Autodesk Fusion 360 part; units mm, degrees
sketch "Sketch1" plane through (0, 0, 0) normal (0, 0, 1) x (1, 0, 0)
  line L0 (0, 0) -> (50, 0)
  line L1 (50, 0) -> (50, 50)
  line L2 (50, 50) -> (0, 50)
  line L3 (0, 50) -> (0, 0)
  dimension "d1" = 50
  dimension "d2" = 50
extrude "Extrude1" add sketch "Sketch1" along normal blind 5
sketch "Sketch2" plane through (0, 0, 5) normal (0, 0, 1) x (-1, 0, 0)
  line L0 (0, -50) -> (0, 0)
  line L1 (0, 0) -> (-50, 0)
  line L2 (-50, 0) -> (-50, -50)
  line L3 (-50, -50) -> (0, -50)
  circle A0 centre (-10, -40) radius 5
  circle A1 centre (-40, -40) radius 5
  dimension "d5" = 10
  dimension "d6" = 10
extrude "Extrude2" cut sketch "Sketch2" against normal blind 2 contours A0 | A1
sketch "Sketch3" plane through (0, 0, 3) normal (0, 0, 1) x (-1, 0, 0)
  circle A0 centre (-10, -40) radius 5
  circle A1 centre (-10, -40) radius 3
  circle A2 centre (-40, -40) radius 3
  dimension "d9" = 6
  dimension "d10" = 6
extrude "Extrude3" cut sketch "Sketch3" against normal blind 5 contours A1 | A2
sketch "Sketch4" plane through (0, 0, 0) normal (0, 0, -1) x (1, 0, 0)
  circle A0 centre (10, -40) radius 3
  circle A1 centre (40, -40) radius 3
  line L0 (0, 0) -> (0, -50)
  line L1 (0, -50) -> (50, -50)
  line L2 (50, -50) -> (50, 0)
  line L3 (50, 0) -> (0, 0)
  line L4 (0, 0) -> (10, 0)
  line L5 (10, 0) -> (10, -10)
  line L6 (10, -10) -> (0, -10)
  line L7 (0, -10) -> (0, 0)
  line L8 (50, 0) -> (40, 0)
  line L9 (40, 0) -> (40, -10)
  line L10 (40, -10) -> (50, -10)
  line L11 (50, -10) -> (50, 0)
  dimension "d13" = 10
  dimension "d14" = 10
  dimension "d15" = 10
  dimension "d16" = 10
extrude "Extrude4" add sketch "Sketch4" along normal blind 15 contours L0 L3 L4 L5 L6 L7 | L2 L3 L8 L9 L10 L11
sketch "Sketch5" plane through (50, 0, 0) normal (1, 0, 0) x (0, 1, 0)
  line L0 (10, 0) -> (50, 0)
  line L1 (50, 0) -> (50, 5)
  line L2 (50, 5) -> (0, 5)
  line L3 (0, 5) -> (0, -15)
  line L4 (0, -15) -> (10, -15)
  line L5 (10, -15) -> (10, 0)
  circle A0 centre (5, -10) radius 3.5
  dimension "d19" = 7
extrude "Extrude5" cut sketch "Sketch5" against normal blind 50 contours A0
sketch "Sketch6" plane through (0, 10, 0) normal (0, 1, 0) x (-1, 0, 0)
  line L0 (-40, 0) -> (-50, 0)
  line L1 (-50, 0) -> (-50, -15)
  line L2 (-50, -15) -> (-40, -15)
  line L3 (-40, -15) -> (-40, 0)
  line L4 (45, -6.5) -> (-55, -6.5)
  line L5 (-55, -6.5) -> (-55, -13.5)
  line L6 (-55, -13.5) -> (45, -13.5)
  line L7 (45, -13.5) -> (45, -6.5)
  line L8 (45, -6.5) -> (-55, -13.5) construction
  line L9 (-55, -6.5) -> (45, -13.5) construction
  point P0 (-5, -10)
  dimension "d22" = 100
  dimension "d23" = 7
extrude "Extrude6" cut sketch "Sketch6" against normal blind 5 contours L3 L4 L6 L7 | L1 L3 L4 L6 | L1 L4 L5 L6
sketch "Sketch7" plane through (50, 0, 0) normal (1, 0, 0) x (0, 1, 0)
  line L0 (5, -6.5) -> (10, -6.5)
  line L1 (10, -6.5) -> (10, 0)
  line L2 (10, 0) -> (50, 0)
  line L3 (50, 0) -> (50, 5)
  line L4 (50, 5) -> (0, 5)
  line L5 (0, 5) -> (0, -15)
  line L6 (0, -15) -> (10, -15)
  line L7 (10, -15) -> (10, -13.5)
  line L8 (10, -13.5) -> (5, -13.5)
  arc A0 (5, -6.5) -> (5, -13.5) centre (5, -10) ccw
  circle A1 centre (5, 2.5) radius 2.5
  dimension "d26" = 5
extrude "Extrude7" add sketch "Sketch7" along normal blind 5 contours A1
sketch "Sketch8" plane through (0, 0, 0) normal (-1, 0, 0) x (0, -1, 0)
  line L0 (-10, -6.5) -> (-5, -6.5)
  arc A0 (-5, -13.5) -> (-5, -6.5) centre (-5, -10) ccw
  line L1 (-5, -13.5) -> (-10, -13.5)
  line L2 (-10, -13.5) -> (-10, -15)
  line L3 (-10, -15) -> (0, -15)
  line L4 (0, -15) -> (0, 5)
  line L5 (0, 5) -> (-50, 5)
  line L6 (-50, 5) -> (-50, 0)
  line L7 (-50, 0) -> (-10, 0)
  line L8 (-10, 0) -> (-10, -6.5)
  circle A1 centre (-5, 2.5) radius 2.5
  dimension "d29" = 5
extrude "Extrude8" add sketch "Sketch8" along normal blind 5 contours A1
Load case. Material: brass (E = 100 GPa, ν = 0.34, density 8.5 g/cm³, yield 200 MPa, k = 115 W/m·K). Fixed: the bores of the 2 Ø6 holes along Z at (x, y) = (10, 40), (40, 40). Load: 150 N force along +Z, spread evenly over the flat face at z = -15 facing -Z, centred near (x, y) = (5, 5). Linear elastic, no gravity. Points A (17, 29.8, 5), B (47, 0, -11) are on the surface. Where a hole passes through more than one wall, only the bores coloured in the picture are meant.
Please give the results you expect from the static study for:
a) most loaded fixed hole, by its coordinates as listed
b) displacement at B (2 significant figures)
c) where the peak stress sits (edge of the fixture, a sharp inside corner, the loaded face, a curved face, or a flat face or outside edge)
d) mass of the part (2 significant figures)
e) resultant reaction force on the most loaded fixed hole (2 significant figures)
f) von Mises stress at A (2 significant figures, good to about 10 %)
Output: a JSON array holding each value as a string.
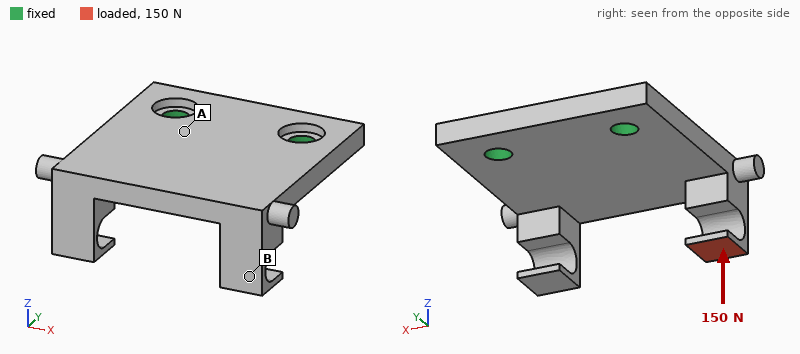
["(10, 40)", "0.050 mm", "a curved face", "120 g", "160 N", "23 MPa"]
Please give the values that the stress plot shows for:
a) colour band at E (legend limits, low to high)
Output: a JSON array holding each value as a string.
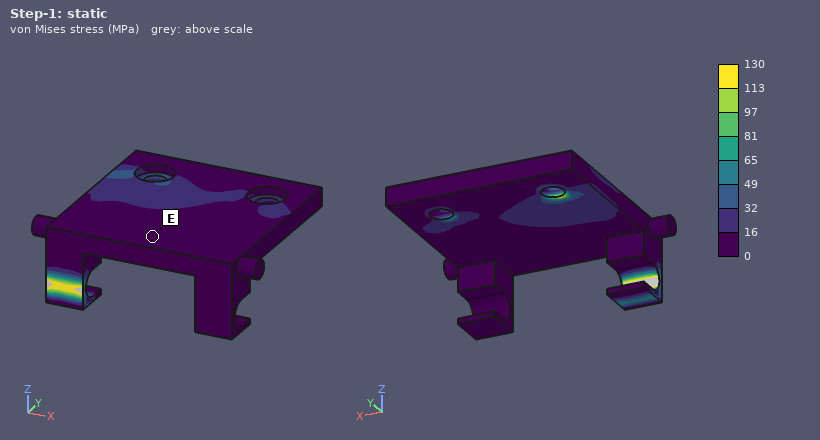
["0 to 16 MPa"]
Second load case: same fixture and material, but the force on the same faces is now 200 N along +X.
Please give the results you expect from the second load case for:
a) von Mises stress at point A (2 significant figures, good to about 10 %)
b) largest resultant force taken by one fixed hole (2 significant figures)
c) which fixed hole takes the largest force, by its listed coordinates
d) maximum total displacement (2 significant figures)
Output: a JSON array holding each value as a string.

["13 MPa", "250 N", "(10, 40)", "0.11 mm"]
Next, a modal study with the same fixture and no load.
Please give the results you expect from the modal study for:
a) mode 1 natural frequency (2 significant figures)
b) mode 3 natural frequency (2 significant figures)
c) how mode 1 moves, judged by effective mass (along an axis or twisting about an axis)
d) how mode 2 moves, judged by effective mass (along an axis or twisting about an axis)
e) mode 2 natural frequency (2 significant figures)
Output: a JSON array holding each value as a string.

["1100 Hz", "4700 Hz", "along Z", "twisting about Y", "2100 Hz"]
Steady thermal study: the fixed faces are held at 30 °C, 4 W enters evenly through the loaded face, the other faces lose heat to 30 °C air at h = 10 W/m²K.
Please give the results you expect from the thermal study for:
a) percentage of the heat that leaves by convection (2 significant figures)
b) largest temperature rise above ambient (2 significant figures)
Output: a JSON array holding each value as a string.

["6.7 %", "32 K"]
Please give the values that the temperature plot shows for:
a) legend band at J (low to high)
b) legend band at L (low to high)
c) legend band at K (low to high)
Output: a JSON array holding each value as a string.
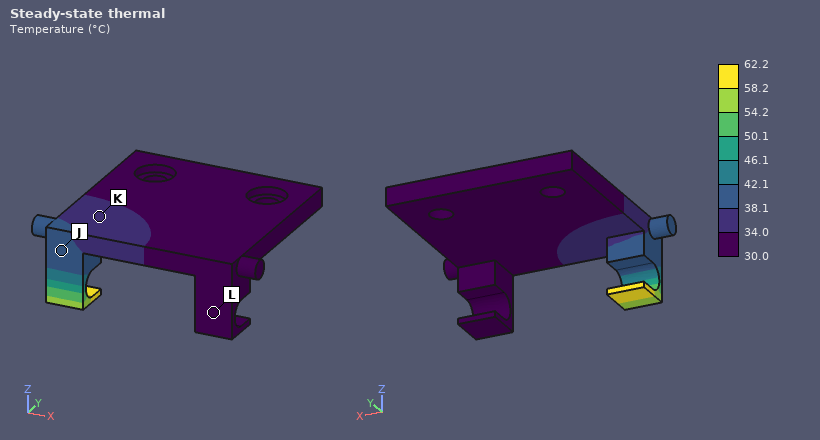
["38.1 to 42.1 °C", "30.0 to 34.0 °C", "34.0 to 38.1 °C"]
